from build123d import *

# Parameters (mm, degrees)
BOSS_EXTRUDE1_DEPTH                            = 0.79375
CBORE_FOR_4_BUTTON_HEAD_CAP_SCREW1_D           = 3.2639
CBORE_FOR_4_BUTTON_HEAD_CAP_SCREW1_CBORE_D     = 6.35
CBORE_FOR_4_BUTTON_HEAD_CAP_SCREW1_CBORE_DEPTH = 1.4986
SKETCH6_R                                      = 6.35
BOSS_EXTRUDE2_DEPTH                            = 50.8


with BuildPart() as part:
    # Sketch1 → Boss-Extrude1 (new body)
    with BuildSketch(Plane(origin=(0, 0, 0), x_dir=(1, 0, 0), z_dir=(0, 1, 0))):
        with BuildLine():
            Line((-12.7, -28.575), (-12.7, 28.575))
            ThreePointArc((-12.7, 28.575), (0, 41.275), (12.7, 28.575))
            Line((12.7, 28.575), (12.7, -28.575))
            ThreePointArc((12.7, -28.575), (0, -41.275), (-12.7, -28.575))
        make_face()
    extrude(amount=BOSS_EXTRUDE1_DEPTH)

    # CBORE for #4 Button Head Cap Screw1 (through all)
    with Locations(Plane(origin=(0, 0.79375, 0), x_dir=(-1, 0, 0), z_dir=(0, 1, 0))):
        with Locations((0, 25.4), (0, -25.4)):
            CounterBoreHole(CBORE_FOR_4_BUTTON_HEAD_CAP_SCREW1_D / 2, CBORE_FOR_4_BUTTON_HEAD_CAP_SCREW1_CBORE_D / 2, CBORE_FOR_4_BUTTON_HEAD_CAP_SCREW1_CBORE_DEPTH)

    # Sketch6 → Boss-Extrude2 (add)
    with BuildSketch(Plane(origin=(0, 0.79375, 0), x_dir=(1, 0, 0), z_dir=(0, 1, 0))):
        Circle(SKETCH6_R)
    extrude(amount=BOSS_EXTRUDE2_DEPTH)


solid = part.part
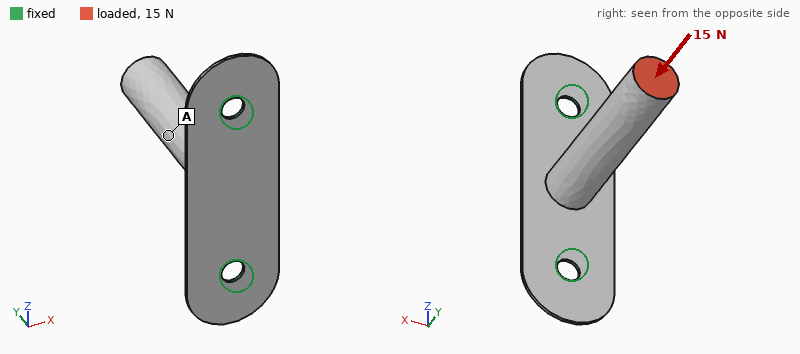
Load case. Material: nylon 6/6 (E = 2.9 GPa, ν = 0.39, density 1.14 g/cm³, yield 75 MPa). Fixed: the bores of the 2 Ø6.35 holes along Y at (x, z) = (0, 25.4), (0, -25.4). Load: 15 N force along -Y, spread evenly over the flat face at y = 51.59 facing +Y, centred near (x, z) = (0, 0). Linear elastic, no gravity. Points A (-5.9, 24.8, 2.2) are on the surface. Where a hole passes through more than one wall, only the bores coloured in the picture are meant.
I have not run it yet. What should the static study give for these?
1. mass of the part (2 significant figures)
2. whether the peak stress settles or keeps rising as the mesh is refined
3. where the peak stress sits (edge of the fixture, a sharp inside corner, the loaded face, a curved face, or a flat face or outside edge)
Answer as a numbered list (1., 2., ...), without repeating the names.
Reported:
1. 9.1 g
2. keeps rising
3. edge of the fixture
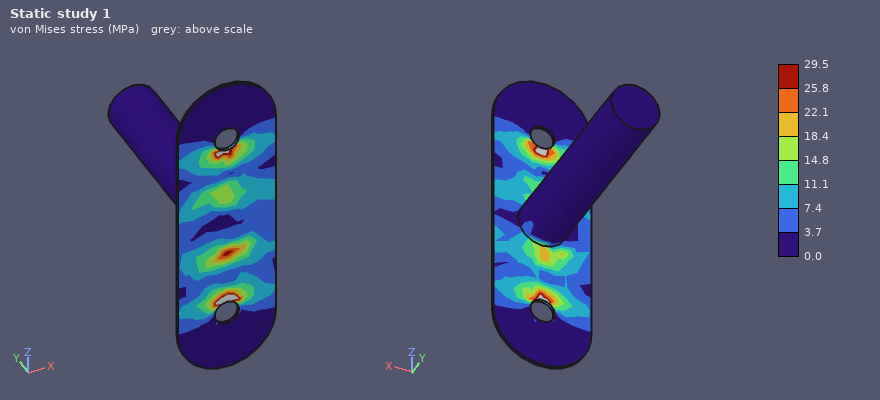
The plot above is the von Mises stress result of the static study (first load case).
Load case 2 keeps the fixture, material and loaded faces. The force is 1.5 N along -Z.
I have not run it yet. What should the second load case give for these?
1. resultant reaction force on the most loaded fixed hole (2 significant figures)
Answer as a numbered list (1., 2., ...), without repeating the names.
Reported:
1. 2.4 N
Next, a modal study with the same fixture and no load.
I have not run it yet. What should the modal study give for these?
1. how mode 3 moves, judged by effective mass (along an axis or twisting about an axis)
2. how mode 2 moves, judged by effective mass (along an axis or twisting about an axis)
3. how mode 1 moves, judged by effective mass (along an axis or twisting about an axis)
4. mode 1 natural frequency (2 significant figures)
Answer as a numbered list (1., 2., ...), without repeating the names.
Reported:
1. along Y
2. along Z
3. along X
4. 53 Hz
